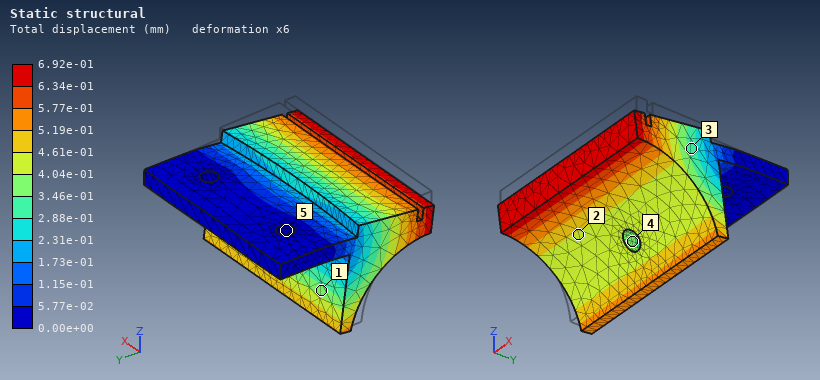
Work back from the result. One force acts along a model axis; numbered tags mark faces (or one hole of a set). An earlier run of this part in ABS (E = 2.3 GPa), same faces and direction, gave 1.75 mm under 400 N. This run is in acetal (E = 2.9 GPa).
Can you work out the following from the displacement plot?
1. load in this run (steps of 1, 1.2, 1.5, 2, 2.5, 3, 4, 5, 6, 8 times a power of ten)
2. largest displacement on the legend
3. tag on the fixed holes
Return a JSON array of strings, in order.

["200 N", "6.92e-01 mm", "5"]
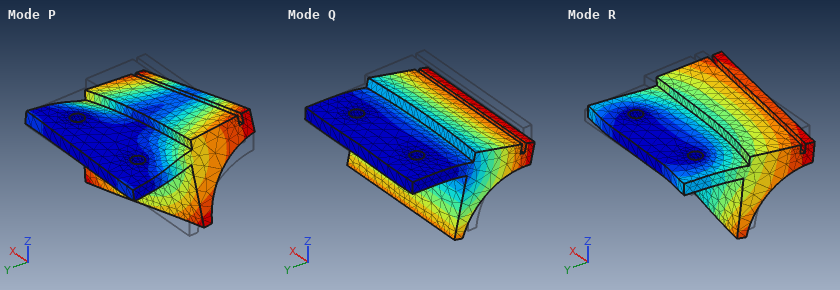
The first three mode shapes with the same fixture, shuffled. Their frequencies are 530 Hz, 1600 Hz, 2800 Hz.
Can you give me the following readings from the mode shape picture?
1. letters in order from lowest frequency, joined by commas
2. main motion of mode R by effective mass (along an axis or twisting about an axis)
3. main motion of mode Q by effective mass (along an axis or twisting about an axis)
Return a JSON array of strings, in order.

["Q, P, R", "along X", "along Z"]
